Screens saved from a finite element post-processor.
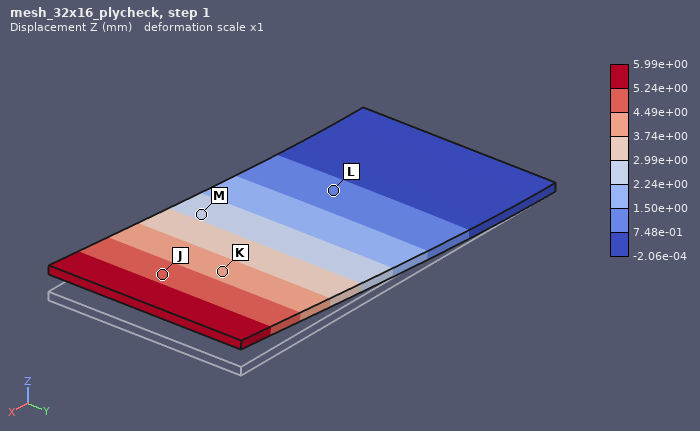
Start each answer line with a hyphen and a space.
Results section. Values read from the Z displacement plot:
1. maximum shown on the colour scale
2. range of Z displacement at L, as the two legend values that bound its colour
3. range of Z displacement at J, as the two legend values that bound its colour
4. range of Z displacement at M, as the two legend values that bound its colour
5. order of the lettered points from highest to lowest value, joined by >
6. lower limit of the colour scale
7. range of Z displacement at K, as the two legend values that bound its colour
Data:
- 5.99e+00 mm
- 7.48e-01 to 1.50e+00 mm
- 4.49e+00 to 5.24e+00 mm
- 2.24e+00 to 2.99e+00 mm
- J > K > M > L
- -2.06e-04 mm
- 3.74e+00 to 4.49e+00 mm
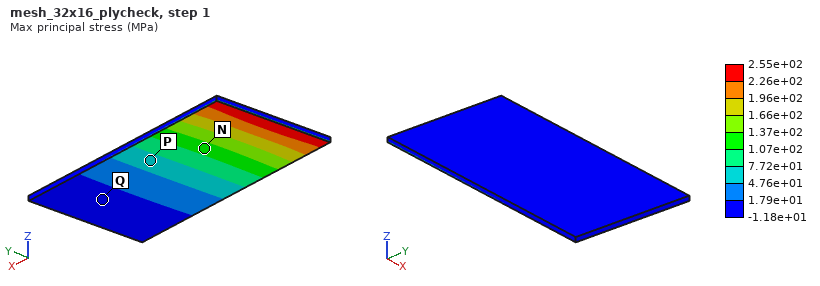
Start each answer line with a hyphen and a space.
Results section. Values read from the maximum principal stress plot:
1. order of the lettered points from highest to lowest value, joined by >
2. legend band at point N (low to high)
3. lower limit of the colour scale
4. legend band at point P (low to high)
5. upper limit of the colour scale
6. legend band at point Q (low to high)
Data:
- N > P > Q
- 1.07e+02 to 1.37e+02 MPa
- -1.18e+01 MPa
- 4.76e+01 to 7.72e+01 MPa
- 2.55e+02 MPa
- -1.18e+01 to 1.79e+01 MPa
